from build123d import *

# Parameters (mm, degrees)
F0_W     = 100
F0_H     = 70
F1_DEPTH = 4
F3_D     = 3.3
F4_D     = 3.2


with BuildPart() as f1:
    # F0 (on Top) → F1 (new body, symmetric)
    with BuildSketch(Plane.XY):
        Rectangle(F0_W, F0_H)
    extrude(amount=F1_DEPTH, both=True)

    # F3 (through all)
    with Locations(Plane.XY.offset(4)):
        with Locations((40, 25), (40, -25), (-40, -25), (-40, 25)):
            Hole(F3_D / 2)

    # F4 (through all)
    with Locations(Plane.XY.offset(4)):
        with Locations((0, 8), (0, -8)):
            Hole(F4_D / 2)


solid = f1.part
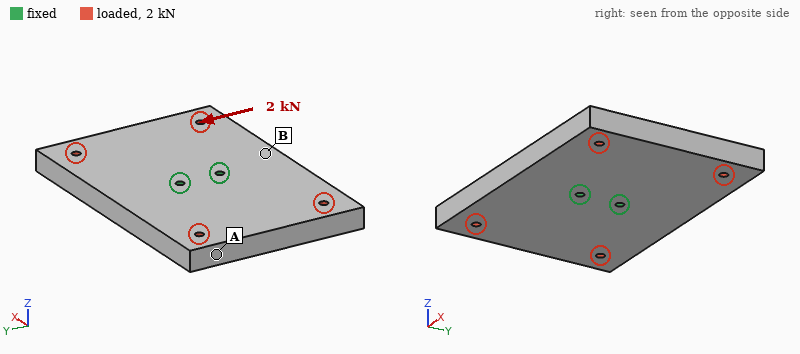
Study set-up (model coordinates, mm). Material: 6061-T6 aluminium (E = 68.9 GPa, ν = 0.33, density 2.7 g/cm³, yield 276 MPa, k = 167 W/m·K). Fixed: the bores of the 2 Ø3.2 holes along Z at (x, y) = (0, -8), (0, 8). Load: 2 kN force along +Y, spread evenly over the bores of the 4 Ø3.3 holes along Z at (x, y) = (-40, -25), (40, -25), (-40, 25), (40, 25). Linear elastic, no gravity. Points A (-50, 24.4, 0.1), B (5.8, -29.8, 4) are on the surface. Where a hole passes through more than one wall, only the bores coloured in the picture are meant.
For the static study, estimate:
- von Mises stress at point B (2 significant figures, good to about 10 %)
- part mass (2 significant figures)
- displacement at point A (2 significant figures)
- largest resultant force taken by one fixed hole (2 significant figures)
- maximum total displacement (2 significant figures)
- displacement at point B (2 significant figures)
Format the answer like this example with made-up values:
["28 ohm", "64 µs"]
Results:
["5.1 MPa", "150 g", "6.2 µm", "1.0 kN", "6.4 µm", "1.6 µm"]
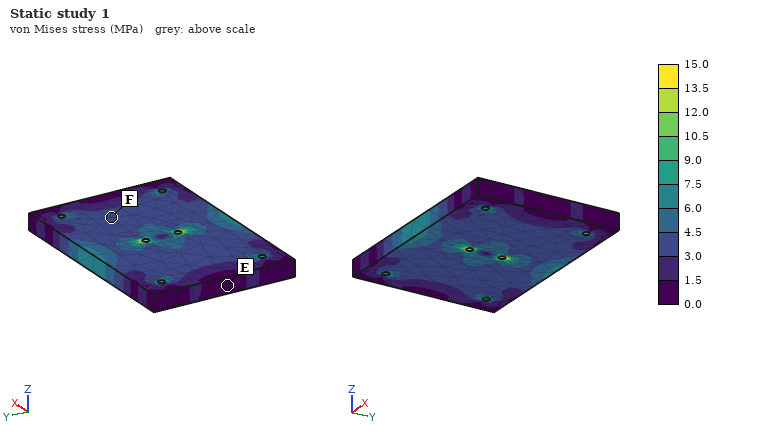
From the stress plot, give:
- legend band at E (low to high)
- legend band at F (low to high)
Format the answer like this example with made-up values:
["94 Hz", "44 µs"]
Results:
["0.0 to 1.5 MPa", "3.0 to 4.5 MPa"]
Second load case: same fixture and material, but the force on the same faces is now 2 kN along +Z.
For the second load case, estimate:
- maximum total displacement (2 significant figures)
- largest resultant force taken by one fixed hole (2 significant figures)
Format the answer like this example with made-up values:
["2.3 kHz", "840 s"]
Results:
["0.14 mm", "1.0 kN"]
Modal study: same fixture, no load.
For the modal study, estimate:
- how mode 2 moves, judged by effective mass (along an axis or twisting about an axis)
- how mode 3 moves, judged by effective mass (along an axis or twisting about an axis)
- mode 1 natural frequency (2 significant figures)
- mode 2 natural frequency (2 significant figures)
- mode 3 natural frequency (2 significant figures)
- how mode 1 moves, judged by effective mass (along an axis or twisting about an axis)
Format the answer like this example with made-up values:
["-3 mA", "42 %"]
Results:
["along Z", "twisting about X", "1800 Hz", "2700 Hz", "3500 Hz", "twisting about Y"]
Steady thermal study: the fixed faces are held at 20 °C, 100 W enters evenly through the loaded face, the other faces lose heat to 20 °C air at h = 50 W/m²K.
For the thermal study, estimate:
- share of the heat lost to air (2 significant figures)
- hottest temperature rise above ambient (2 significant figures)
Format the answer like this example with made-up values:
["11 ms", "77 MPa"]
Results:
["17 %", "33 K"]
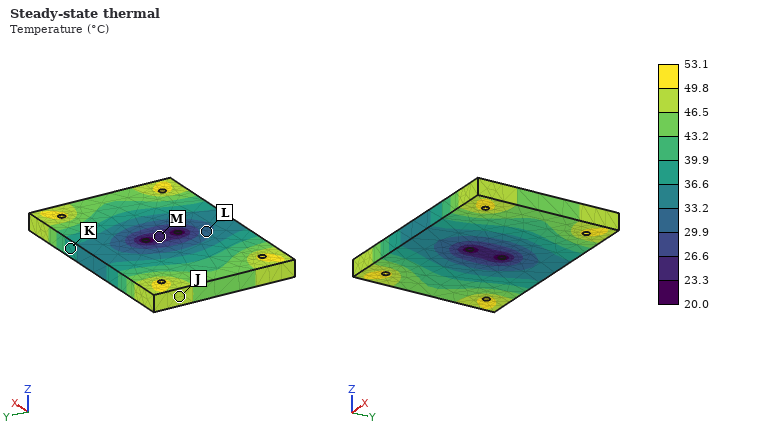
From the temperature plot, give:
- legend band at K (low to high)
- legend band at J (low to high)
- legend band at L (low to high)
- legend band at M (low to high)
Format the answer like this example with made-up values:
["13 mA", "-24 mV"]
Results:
["36.6 to 39.9 °C", "46.5 to 49.8 °C", "29.9 to 33.2 °C", "23.3 to 26.6 °C"]
